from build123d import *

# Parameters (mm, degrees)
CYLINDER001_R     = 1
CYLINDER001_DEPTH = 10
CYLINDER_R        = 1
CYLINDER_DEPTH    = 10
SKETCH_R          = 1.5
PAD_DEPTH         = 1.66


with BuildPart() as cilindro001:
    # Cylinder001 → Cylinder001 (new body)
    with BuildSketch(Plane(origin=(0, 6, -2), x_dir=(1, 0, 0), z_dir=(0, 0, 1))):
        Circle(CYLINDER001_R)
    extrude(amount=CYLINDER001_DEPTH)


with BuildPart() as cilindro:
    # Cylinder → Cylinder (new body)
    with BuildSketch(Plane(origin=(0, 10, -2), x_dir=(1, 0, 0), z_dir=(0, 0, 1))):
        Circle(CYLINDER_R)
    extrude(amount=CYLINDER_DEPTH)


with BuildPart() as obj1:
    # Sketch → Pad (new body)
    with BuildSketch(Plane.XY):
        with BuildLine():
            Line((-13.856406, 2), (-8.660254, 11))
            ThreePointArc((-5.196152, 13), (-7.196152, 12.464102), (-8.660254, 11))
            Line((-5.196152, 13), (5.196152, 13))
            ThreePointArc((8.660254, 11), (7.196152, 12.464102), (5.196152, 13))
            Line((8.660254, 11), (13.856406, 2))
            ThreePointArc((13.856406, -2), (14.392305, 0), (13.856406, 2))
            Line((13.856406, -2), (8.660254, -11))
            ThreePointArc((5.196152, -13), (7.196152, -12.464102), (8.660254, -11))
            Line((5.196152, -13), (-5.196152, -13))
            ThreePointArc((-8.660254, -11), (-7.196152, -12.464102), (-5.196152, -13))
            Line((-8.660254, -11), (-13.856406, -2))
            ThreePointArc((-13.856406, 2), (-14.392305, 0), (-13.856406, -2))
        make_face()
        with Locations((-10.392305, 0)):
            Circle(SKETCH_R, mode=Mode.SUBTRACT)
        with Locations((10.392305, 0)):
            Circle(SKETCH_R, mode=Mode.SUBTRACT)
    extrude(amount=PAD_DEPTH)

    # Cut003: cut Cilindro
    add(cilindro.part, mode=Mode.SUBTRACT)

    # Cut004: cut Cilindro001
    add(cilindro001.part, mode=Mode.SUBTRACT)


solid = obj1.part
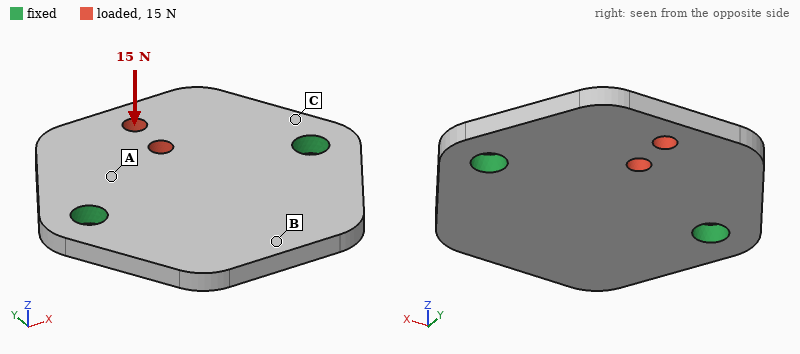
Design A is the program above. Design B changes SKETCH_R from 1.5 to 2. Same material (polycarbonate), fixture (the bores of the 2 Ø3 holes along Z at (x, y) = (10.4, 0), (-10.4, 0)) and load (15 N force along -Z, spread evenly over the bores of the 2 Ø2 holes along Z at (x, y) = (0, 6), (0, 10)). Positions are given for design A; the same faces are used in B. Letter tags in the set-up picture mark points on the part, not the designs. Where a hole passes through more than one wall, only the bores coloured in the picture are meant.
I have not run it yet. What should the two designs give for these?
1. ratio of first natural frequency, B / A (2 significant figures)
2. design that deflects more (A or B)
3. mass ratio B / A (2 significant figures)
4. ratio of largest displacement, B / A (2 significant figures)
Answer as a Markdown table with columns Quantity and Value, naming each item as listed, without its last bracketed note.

| Quantity | Value |
|---|---|
| ratio of first natural frequency, B / A | 1.1 |
| design that deflects more | A |
| mass ratio B / A | 0.98 |
| ratio of largest displacement, B / A | 0.86 |
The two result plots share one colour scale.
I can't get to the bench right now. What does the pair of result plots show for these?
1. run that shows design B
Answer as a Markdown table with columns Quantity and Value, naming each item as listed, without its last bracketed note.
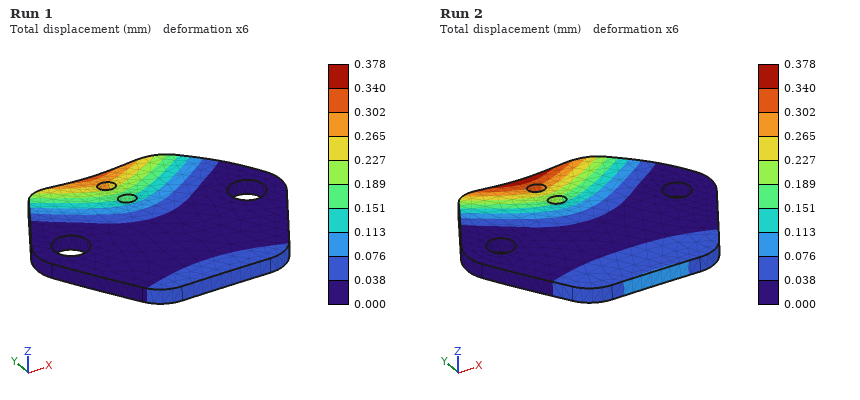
| Quantity | Value |
|---|---|
| run that shows design B | Run 1 |
